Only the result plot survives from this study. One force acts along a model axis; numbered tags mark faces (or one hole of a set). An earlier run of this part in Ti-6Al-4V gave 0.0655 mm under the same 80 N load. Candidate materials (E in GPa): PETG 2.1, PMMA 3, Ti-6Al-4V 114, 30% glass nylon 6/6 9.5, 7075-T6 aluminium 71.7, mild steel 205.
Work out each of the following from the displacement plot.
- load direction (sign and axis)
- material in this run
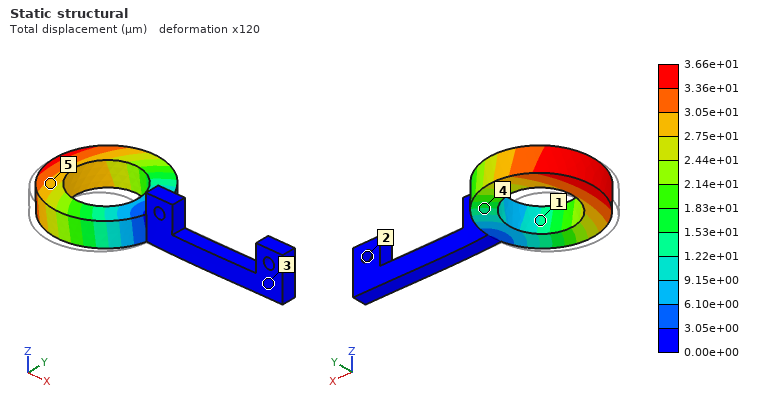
+Y
mild steel
